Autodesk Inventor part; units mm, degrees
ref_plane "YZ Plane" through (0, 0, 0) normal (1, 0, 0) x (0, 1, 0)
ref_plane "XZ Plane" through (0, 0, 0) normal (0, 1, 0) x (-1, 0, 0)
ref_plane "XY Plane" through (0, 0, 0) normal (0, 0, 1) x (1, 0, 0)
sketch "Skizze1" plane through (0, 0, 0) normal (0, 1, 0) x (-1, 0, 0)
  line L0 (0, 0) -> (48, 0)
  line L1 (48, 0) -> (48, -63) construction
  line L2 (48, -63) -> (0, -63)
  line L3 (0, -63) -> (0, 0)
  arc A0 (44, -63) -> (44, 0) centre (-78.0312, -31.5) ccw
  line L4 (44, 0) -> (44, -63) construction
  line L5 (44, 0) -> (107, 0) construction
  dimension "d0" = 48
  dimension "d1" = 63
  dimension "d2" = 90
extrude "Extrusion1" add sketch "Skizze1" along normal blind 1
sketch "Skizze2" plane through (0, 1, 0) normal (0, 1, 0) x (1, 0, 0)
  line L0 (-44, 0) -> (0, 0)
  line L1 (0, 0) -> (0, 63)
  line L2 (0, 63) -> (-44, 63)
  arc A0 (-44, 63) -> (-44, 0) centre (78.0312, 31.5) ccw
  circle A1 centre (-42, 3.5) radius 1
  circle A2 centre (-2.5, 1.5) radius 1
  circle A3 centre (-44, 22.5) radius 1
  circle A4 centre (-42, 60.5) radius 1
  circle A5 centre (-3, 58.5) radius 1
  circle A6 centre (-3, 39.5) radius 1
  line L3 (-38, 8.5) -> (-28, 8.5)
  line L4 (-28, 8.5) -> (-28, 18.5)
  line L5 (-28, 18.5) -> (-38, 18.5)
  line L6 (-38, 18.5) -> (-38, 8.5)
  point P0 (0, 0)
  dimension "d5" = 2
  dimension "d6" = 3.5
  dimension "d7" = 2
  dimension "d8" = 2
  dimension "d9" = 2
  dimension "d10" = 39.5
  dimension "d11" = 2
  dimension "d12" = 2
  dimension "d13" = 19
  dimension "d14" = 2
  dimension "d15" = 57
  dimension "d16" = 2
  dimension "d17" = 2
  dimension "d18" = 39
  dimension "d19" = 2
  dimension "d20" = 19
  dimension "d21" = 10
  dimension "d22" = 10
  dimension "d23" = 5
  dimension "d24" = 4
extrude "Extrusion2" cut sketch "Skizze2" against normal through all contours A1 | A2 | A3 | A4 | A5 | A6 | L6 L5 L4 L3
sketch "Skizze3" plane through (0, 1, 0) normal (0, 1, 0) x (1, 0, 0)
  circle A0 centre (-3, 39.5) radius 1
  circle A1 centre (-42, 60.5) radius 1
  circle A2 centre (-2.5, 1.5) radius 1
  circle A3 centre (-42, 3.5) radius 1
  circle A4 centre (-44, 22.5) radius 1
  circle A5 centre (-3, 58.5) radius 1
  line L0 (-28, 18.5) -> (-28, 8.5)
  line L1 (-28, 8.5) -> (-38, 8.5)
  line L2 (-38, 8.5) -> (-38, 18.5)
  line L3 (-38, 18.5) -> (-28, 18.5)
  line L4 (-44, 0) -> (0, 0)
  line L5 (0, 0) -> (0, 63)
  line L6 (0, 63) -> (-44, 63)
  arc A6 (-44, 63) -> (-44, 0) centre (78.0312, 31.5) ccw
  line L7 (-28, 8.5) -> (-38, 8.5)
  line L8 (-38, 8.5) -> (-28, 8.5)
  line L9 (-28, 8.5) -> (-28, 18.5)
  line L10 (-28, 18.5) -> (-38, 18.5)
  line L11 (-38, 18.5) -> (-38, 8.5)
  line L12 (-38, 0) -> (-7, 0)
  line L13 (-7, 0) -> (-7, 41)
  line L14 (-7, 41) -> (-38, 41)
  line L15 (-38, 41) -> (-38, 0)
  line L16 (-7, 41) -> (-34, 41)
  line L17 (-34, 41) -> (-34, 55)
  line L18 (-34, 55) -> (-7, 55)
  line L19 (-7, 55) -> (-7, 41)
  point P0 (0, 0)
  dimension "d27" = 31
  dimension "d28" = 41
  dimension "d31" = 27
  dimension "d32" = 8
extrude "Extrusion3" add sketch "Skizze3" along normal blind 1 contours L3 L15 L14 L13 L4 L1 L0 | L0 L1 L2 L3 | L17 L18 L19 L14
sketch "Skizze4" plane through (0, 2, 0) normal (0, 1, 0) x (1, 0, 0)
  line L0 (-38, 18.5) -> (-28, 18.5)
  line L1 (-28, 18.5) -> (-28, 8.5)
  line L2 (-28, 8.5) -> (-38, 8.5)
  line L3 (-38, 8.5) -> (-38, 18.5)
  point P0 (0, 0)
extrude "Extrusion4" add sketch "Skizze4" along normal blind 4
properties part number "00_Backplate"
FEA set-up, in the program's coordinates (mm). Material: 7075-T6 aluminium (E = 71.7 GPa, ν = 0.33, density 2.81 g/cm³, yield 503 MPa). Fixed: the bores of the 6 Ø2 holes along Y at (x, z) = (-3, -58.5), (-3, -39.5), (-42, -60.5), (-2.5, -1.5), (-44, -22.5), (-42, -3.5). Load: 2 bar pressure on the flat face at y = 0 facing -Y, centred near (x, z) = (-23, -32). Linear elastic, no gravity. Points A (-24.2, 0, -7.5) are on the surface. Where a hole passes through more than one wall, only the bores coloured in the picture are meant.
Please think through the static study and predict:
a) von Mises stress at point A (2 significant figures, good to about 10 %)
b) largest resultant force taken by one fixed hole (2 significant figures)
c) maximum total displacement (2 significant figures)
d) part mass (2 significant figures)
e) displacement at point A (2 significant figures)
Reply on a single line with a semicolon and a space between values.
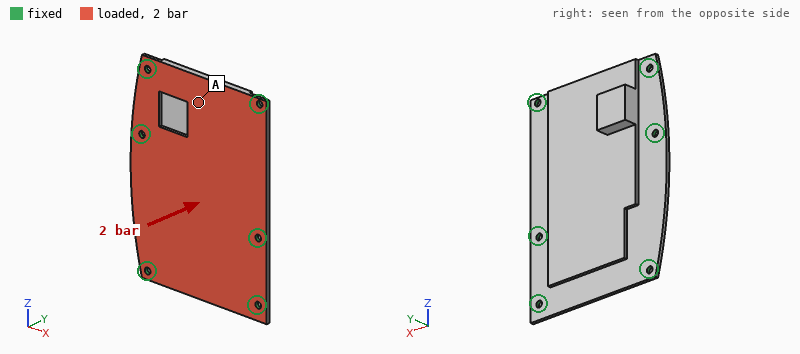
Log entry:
26 MPa; 290 N; 0.15 mm; 14 g; 0.074 mm
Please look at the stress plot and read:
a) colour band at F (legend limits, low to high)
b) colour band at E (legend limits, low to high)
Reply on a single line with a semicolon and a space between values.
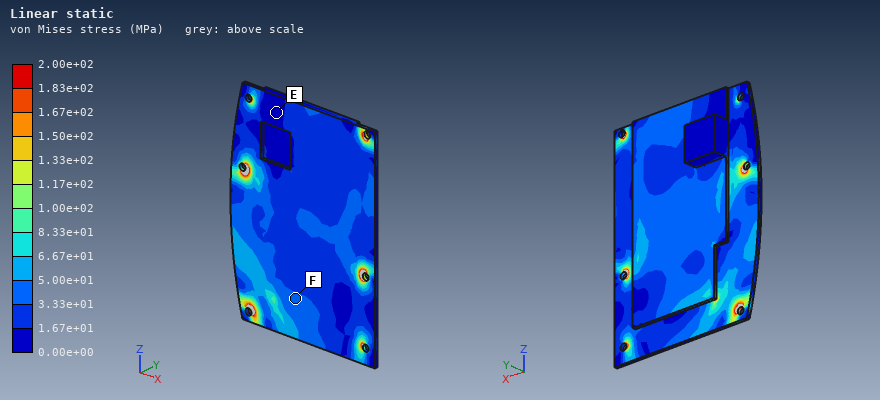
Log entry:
3.33e+01 to 5.00e+01 MPa; 0.00e+00 to 1.67e+01 MPa
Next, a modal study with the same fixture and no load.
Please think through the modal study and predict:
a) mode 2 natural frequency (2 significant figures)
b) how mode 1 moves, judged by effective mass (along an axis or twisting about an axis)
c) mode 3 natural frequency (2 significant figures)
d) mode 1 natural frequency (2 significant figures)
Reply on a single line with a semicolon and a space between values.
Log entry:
4000 Hz; along Y; 5400 Hz; 3100 Hz
